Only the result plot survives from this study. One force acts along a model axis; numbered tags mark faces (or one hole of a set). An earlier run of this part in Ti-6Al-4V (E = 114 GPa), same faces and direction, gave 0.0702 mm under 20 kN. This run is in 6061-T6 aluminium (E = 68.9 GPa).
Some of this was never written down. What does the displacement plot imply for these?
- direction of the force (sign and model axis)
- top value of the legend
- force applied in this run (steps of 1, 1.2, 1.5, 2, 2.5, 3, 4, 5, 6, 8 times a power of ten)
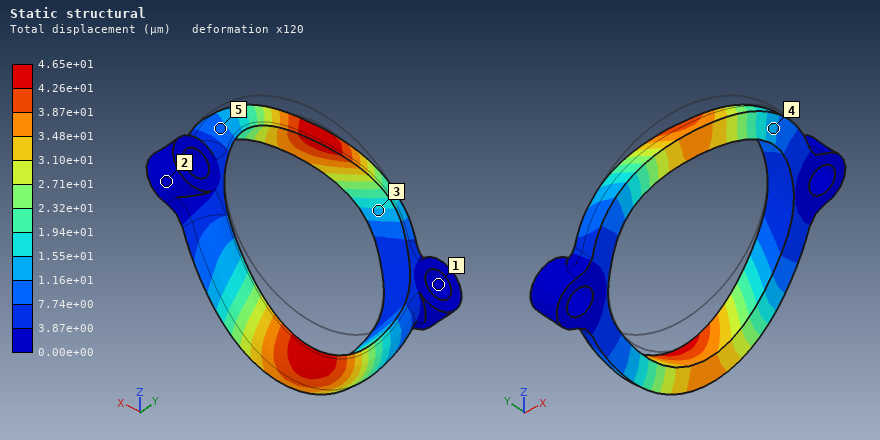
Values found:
-Z
4.65e+01 µm
8 kN
